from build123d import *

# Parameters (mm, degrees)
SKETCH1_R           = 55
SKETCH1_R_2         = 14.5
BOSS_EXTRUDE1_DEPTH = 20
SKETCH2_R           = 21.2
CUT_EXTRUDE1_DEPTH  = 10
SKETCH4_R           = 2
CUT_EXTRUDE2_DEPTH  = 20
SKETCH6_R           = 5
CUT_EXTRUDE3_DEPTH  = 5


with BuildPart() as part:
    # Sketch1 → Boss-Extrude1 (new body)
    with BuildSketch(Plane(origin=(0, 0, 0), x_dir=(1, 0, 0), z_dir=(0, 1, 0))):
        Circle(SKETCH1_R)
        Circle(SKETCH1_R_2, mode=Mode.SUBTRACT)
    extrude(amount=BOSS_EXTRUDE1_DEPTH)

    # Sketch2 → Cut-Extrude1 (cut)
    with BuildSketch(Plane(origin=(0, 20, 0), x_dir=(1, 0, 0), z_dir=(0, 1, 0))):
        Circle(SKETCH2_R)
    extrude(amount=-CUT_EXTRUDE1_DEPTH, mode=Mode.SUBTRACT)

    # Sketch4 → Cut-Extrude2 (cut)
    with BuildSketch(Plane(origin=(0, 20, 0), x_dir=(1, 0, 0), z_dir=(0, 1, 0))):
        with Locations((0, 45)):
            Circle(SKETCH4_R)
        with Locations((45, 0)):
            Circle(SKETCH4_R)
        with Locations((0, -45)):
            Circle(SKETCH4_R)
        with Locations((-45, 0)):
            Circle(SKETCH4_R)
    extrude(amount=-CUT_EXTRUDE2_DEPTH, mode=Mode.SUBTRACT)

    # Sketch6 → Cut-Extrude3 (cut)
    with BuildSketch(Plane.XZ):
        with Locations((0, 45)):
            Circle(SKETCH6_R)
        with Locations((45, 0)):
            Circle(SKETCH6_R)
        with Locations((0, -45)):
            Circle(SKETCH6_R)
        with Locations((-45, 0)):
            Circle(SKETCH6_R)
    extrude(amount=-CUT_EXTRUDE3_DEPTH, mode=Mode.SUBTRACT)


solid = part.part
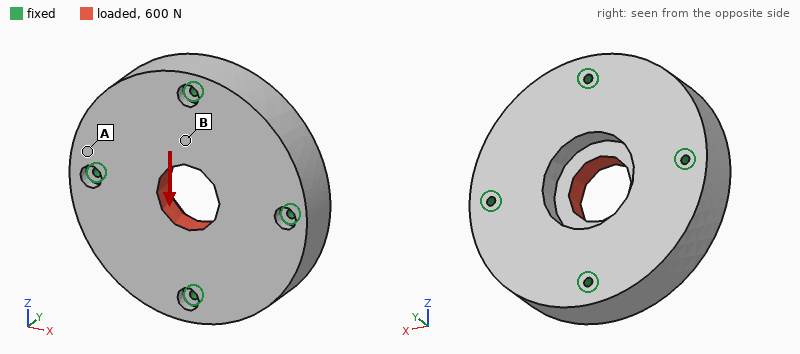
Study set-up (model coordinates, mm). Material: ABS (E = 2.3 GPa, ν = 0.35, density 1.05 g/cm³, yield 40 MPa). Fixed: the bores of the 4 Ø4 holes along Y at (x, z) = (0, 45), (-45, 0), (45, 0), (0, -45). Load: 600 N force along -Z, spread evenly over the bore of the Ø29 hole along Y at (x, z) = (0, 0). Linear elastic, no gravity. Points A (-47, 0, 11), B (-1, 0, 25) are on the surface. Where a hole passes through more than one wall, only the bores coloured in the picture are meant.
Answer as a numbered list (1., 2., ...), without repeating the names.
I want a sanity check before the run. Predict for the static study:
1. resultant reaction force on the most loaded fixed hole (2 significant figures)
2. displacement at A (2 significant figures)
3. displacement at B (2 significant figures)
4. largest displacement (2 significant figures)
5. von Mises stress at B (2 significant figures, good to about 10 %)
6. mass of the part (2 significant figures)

1. 180 N
2. 3.2 µm
3. 8.1 µm
4. 12 µm
5. 0.77 MPa
6. 180 g
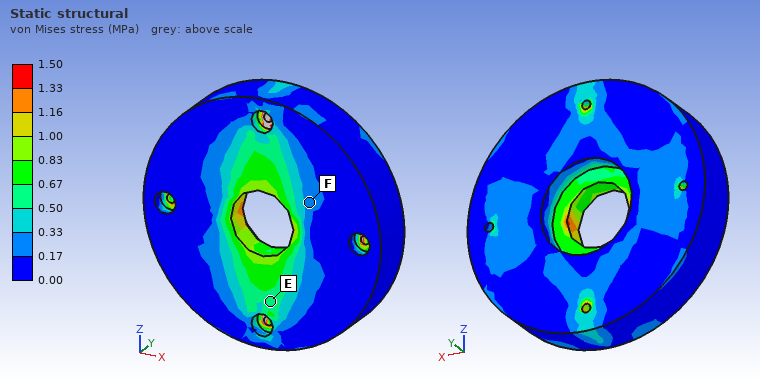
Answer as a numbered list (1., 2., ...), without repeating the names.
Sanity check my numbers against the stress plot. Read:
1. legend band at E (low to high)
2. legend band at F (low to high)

1. 0.50 to 0.67 MPa
2. 0.17 to 0.33 MPa
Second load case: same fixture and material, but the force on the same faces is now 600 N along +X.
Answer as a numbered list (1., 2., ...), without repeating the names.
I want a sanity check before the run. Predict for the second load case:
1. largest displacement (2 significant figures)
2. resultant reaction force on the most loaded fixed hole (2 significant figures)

1. 12 µm
2. 180 N
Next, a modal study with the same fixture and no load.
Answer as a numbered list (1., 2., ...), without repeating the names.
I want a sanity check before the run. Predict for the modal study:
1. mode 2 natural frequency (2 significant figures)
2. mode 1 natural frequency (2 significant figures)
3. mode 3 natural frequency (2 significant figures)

1. 3200 Hz
2. 2900 Hz
3. 3300 Hz
